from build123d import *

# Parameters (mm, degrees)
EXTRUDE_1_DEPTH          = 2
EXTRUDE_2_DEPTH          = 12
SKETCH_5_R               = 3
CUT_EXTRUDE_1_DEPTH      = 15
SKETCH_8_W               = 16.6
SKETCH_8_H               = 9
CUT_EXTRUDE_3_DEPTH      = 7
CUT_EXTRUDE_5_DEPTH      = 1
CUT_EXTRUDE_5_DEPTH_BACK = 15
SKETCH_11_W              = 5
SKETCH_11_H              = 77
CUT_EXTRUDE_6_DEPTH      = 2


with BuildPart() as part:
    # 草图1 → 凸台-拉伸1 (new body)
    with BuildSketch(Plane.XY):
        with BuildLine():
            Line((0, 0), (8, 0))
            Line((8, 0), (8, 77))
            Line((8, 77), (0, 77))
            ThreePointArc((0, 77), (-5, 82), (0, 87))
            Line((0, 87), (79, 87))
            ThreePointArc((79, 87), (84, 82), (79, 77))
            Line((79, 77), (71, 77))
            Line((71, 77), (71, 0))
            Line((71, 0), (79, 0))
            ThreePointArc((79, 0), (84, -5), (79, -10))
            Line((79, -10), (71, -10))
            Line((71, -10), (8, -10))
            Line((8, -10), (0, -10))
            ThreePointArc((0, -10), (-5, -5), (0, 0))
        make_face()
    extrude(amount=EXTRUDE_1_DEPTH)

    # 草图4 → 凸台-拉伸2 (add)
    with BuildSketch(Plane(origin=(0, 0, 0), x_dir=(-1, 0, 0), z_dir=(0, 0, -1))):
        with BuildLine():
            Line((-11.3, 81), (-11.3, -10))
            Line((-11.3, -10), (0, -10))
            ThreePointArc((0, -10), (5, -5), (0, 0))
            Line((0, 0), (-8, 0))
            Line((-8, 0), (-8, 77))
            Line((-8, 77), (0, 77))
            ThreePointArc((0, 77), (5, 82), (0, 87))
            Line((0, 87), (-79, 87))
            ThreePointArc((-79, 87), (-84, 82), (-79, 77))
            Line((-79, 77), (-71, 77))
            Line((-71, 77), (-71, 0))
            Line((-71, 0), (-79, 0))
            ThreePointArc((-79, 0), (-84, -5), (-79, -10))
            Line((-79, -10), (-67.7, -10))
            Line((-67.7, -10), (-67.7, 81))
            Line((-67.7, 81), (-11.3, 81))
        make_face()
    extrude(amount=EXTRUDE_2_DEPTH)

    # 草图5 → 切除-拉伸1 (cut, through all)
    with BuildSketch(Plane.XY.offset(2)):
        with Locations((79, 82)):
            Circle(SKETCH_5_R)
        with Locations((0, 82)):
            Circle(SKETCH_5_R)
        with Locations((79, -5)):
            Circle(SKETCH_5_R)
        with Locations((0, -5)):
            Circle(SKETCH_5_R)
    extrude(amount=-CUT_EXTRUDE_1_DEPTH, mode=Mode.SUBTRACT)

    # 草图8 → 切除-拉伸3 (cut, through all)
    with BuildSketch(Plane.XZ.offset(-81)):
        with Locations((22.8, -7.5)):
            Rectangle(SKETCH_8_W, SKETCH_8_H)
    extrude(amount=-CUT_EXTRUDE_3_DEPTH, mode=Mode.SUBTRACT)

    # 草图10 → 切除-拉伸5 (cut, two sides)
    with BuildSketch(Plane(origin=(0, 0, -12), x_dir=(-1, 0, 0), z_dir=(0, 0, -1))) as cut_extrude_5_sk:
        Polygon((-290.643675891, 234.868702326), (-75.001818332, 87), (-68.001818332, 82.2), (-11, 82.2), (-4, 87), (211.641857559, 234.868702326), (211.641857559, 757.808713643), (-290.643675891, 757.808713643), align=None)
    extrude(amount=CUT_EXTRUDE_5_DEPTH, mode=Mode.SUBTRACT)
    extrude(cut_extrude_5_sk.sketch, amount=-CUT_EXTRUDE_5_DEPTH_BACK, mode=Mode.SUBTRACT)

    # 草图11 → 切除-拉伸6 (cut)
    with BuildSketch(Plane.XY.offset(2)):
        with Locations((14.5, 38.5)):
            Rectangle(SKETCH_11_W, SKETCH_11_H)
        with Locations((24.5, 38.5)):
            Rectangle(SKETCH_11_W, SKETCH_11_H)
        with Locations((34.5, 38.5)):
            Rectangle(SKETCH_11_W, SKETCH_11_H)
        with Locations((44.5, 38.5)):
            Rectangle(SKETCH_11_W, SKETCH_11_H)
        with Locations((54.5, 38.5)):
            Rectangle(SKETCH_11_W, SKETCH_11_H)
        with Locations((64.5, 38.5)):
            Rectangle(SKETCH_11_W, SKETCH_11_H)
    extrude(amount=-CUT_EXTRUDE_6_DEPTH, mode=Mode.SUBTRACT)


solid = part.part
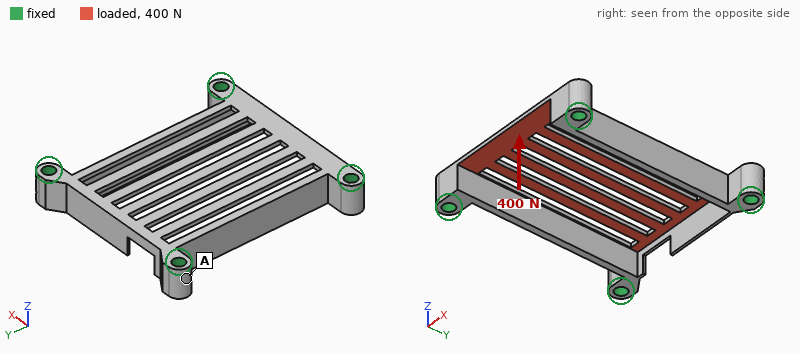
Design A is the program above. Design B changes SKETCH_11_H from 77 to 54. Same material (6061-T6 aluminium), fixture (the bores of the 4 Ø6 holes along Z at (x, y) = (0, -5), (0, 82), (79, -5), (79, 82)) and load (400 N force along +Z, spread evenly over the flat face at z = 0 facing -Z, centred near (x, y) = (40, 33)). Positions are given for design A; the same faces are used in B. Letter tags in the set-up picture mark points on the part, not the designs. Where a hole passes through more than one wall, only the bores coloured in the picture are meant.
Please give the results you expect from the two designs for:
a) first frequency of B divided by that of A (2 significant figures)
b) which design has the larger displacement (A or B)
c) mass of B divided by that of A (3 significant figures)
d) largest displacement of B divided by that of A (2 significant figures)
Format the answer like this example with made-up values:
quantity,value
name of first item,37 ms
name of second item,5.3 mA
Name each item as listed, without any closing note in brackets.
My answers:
quantity,value
first frequency of B divided by that of A,1.6
which design has the larger displacement,A
mass of B divided by that of A,1.07
largest displacement of B divided by that of A,0.33
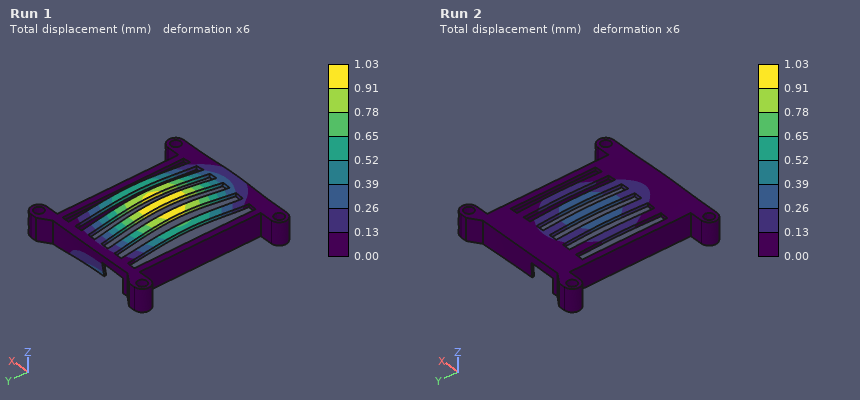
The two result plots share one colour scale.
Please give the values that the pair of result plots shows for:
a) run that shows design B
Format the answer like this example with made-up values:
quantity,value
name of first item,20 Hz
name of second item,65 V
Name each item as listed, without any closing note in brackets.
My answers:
quantity,value
run that shows design B,Run 2
